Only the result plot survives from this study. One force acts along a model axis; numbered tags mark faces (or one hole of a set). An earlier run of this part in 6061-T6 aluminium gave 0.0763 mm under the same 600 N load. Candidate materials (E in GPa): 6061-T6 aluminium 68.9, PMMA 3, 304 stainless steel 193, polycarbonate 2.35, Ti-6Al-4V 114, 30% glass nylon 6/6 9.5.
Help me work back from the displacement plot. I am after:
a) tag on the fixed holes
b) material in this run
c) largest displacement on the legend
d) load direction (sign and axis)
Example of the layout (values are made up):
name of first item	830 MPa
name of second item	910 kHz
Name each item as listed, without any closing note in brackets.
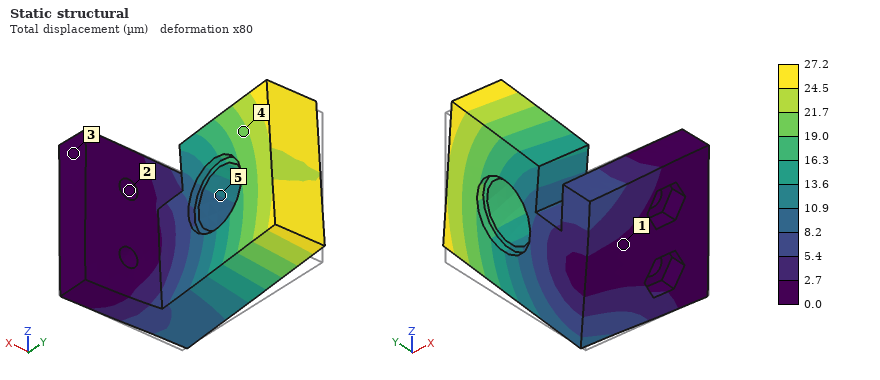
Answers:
tag on the fixed holes	2
material in this run	304 stainless steel
largest displacement on the legend	27.2 µm
load direction	+Z
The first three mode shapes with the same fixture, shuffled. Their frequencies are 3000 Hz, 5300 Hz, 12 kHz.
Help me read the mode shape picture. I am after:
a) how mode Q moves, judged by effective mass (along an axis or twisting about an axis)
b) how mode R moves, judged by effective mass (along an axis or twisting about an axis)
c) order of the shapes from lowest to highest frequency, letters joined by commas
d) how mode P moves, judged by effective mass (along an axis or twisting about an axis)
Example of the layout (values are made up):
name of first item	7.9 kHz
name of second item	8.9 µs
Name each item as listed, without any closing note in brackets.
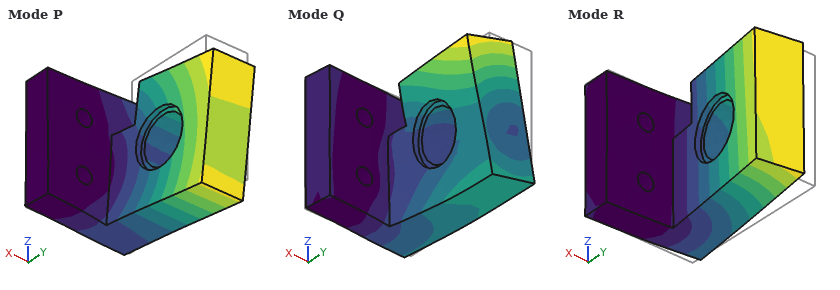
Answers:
how mode Q moves, judged by effective mass	along Y
how mode R moves, judged by effective mass	along X
order of the shapes from lowest to highest frequency, letters joined by commas	R, P, Q
how mode P moves, judged by effective mass	along Z
